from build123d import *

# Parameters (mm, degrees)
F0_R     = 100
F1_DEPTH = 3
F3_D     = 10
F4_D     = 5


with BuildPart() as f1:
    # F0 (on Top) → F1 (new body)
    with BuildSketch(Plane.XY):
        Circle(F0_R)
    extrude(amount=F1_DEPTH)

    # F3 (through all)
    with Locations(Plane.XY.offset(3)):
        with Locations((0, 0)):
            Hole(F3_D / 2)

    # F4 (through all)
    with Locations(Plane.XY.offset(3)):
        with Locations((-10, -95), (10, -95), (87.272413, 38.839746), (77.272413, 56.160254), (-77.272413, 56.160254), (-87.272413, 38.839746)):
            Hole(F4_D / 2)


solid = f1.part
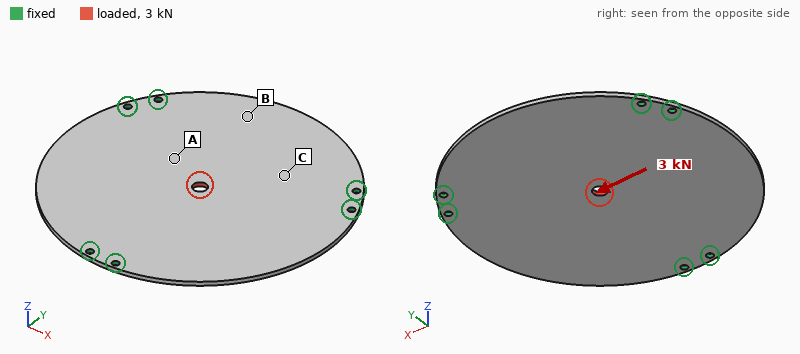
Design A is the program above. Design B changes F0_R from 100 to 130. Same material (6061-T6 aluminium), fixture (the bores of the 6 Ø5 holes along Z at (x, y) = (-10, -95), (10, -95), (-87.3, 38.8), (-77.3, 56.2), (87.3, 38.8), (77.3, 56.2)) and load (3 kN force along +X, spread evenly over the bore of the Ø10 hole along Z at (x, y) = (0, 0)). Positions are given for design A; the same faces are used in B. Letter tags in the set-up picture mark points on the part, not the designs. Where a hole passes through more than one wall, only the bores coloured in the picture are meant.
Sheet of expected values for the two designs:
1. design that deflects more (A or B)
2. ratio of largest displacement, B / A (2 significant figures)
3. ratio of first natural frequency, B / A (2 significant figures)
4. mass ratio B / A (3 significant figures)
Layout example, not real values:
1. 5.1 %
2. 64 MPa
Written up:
1. A
2. 0.88
3. 0.76
4. 1.69
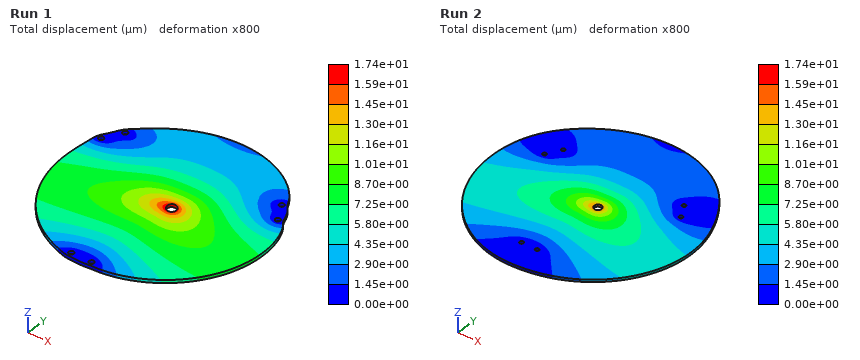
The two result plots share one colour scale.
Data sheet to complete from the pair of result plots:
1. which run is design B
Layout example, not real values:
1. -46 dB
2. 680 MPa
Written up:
1. Run 2
